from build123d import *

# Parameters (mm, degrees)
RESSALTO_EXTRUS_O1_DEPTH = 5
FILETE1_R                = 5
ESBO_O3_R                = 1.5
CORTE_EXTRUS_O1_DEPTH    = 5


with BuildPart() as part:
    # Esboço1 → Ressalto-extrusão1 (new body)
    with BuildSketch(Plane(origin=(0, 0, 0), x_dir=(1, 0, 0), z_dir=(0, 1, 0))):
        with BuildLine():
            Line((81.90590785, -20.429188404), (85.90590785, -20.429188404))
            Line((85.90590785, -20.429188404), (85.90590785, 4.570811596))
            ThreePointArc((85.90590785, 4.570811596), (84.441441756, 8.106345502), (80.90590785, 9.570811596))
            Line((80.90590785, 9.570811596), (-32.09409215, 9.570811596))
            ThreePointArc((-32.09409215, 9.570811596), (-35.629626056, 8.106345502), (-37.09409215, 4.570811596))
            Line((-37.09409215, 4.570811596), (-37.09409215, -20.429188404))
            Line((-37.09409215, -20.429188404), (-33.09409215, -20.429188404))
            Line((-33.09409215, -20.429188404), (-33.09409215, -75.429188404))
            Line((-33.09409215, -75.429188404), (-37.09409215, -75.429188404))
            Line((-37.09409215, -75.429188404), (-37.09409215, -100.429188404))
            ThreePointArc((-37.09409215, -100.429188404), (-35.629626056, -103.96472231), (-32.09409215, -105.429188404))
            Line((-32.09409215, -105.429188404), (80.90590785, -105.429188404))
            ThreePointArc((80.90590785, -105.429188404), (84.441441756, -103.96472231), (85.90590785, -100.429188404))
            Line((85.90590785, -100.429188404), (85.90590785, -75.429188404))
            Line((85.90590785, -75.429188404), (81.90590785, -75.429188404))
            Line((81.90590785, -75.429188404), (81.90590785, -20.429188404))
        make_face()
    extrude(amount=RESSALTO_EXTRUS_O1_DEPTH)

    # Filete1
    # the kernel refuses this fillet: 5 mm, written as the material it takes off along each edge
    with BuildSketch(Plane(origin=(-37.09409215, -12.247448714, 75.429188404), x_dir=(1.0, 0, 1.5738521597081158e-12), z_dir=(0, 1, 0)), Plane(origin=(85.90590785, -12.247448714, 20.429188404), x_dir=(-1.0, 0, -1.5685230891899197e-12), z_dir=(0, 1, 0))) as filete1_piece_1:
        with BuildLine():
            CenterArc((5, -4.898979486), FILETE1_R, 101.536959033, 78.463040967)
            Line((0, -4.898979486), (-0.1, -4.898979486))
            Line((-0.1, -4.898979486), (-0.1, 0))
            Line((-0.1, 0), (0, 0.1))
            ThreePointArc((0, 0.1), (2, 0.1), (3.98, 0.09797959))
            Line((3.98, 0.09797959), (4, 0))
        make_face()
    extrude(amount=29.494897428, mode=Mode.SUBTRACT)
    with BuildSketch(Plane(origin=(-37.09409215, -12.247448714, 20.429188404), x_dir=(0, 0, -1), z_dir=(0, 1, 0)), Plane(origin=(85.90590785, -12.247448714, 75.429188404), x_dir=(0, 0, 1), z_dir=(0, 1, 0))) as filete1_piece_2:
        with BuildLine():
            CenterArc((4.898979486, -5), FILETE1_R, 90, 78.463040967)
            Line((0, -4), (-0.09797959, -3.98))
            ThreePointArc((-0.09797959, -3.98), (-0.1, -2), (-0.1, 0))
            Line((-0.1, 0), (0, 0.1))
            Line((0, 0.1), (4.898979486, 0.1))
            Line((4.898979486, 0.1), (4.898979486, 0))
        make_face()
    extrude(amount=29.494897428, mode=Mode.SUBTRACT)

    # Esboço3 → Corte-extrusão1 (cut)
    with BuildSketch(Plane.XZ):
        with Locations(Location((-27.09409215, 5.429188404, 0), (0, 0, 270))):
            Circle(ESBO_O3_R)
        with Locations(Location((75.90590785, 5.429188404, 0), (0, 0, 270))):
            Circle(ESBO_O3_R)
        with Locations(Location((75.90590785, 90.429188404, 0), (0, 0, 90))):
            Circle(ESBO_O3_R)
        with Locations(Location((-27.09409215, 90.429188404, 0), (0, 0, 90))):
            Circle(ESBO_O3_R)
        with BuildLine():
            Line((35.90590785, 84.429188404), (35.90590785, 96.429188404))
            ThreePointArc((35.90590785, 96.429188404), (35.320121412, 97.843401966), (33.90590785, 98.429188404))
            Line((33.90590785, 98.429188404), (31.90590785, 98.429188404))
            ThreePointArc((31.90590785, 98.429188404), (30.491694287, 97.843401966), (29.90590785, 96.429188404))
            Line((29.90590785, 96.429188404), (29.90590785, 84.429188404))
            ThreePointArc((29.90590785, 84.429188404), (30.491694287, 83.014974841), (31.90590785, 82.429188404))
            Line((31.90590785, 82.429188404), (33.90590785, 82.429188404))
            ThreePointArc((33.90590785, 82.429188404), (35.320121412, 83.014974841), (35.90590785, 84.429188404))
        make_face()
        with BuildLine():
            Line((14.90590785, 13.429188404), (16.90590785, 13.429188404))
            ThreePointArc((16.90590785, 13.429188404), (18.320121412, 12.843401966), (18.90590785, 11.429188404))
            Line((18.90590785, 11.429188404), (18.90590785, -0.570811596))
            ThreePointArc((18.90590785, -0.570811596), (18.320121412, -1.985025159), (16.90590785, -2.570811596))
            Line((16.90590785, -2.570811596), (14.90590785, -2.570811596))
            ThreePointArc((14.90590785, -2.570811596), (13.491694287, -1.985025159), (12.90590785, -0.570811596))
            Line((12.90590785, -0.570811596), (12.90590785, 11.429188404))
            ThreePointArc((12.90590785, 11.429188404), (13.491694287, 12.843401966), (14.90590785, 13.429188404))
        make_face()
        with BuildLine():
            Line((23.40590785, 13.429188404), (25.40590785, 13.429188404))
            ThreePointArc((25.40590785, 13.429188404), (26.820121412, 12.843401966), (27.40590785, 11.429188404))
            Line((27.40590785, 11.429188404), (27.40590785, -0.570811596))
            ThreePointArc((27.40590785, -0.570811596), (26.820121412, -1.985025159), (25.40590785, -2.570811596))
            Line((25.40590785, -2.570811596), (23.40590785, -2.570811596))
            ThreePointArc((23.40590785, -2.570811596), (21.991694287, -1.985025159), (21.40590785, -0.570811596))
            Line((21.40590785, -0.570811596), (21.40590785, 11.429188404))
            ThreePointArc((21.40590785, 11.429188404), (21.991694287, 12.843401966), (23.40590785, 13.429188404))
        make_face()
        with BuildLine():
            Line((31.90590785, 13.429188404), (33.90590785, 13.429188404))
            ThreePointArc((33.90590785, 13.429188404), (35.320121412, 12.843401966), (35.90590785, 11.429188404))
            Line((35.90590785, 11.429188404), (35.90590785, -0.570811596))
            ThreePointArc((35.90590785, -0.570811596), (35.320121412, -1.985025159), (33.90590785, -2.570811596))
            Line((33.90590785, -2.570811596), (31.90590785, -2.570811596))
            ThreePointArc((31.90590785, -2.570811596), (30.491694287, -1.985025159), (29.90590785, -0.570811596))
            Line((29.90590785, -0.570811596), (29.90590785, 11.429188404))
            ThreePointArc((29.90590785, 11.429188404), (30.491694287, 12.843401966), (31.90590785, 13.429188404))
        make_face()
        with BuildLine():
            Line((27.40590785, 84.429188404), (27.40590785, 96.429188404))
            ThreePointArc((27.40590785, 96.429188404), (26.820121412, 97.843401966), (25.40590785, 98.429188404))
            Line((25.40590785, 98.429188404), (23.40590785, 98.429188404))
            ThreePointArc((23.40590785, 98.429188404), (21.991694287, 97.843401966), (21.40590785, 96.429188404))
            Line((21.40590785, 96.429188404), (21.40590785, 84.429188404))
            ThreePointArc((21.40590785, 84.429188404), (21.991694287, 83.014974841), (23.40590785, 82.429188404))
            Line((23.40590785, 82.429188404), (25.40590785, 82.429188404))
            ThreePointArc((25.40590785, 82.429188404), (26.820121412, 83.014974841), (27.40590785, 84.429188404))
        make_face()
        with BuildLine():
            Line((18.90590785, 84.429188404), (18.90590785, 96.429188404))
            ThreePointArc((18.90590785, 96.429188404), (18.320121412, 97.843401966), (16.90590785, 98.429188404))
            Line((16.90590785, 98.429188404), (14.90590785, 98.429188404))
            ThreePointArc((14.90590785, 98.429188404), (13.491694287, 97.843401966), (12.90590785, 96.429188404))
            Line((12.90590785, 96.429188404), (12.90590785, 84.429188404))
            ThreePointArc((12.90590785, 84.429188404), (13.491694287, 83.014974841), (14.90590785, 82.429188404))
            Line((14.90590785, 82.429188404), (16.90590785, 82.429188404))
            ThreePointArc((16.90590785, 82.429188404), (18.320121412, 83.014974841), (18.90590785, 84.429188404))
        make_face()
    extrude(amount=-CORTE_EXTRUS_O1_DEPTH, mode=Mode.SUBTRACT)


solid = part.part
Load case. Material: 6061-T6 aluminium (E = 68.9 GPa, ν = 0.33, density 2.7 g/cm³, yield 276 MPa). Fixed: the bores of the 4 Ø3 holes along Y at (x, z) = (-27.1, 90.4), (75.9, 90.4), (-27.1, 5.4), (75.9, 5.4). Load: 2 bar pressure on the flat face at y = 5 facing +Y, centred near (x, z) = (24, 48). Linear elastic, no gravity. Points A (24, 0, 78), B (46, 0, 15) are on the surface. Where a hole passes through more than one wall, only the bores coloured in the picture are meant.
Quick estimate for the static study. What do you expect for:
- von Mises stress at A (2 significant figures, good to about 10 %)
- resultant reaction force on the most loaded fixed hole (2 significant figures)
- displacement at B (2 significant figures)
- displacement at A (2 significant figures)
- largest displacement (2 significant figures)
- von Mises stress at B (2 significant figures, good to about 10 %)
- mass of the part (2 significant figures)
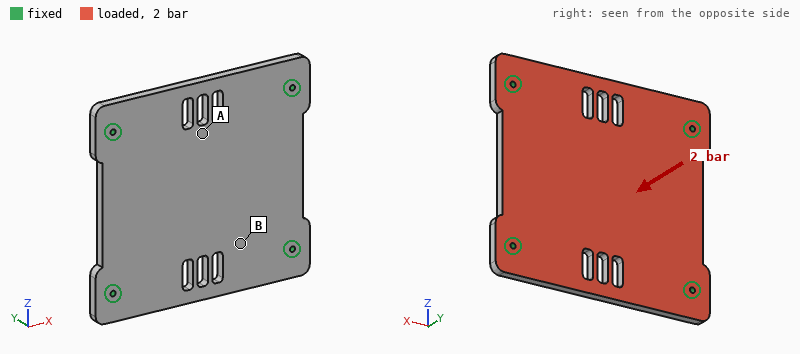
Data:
33 MPa
650 N
0.12 mm
0.17 mm
0.19 mm
15 MPa
180 g
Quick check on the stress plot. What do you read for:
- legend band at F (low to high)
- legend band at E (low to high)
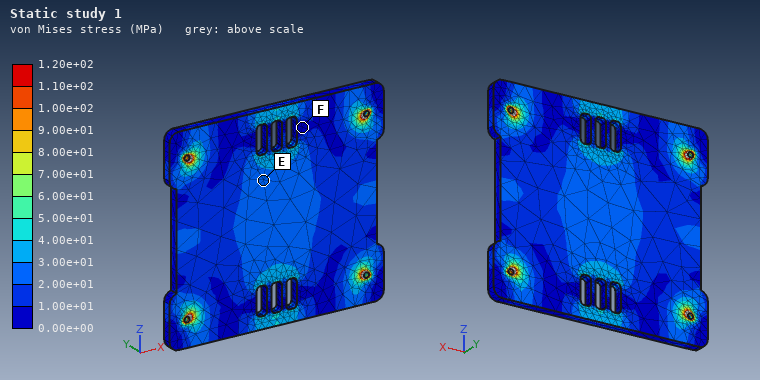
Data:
0.00e+00 to 1.00e+01 MPa
2.00e+01 to 3.00e+01 MPa
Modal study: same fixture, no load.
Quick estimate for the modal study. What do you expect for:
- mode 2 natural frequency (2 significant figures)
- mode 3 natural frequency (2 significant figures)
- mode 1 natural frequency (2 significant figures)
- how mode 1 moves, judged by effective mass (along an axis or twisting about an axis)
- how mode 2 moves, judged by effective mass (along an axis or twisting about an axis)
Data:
2500 Hz
3200 Hz
1700 Hz
along Y
twisting about X
